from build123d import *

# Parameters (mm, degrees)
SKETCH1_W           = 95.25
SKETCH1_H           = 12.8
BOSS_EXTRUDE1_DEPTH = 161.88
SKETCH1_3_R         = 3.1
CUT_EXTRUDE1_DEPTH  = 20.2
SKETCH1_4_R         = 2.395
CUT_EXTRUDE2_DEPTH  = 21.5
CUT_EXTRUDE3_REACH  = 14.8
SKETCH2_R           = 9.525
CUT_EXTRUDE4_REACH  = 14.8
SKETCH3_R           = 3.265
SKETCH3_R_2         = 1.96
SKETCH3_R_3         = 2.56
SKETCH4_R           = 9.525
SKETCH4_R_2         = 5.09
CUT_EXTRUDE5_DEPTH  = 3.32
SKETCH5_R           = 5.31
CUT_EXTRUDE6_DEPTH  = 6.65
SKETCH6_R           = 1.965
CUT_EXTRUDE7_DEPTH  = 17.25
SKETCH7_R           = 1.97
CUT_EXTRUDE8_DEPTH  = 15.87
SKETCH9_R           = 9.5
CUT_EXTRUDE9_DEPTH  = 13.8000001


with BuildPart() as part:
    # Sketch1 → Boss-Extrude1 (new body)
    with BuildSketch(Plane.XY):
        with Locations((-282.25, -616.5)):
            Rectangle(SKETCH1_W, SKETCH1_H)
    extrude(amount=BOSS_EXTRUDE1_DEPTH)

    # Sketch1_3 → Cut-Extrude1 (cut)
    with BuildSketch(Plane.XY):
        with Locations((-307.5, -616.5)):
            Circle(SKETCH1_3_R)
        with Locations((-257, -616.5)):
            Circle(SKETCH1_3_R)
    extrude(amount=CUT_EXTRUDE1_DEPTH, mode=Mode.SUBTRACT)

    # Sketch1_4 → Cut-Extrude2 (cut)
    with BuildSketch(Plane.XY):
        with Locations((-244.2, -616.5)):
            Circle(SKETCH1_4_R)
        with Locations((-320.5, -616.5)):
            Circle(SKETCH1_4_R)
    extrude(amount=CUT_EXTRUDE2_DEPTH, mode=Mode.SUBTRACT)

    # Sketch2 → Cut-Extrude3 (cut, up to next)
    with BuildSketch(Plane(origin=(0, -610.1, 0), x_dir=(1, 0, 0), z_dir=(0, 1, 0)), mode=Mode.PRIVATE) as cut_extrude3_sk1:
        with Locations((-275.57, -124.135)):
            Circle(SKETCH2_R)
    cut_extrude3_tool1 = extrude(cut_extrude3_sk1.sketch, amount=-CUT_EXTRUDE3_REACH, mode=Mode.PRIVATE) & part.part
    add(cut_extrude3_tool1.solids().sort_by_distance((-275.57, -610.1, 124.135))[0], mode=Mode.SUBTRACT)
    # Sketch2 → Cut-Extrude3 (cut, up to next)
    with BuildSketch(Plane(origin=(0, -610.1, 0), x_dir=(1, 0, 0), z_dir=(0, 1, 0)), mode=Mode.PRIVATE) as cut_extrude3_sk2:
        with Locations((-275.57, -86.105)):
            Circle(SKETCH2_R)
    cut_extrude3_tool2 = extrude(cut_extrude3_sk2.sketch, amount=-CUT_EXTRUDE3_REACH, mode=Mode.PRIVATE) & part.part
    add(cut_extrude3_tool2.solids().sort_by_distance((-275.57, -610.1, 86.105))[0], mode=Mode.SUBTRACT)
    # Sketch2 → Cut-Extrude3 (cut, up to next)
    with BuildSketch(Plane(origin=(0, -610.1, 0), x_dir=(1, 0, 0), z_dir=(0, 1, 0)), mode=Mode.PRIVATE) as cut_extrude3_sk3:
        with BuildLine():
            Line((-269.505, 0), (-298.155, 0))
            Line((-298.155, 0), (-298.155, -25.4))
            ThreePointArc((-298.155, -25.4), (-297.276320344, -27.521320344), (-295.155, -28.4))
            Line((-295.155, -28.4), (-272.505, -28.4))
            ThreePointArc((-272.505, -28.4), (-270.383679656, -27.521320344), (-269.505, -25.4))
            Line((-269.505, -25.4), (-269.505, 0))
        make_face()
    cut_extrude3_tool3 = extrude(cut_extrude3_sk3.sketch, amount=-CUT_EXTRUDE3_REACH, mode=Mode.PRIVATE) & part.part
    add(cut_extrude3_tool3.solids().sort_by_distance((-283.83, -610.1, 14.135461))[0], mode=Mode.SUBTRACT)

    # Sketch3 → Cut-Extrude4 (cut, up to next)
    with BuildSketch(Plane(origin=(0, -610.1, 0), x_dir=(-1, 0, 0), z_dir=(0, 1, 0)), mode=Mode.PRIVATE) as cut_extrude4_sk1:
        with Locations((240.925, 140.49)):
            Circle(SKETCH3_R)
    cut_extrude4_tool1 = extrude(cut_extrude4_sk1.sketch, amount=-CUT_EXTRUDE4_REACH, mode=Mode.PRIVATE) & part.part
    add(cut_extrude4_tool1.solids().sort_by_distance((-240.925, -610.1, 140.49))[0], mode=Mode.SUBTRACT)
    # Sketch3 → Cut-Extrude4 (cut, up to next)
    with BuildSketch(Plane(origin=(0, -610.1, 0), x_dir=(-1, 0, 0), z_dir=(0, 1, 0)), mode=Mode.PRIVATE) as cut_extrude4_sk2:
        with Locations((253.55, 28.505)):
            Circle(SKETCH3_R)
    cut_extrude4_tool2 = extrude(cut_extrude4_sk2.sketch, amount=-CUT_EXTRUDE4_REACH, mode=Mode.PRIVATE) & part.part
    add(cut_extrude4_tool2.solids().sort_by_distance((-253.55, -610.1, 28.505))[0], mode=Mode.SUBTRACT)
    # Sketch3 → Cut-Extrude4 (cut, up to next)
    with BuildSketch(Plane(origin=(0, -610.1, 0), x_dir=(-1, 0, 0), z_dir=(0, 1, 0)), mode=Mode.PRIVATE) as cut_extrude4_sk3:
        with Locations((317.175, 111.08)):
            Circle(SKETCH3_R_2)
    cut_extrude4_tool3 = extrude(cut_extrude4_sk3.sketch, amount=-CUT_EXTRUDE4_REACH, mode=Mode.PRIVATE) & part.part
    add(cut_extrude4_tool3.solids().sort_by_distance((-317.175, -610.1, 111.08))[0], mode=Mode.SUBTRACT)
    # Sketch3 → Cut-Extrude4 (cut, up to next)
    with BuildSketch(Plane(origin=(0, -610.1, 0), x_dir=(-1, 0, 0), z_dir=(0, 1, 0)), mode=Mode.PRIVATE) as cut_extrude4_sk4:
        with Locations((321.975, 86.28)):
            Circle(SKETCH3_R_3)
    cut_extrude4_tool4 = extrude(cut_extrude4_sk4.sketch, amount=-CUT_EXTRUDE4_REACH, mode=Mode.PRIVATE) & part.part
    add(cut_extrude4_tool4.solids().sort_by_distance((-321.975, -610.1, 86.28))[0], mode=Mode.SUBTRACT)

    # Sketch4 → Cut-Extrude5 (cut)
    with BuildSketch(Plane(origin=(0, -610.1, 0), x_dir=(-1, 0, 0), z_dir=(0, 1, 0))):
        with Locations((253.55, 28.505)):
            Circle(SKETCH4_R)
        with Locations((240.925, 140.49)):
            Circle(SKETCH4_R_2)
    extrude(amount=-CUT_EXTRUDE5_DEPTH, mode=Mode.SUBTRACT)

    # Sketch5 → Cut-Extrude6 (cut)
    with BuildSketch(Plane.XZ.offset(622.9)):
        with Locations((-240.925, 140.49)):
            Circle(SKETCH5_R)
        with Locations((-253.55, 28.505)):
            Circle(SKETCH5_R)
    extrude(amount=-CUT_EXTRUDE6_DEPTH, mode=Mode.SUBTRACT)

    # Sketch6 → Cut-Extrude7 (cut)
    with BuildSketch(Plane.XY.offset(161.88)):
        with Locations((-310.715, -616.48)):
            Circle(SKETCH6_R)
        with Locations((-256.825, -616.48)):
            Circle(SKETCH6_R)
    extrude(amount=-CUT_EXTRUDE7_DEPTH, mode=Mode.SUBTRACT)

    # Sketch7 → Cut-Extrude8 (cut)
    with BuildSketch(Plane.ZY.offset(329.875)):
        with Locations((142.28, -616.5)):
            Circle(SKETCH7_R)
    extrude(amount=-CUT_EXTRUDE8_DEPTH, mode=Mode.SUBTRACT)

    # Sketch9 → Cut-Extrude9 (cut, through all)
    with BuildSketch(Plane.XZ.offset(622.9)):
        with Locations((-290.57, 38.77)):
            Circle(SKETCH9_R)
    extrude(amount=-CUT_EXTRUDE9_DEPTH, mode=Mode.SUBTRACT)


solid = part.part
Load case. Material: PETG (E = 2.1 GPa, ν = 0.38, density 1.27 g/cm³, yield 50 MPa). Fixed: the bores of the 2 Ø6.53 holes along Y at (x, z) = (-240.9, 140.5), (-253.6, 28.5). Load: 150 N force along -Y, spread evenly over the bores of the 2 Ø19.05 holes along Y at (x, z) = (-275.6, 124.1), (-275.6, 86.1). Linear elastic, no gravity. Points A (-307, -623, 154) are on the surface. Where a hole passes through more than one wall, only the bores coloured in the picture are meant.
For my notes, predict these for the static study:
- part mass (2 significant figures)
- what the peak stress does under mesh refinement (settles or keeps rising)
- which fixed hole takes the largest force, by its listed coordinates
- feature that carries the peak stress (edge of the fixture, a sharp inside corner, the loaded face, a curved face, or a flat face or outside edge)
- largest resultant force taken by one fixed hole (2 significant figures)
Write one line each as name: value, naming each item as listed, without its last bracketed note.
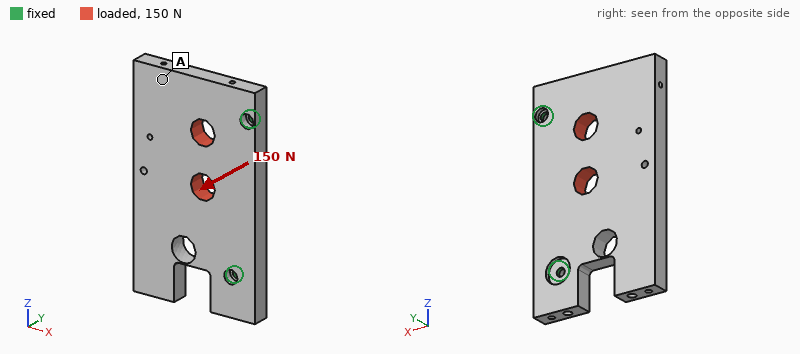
part mass: 220 g
what the peak stress does under mesh refinement: keeps rising
which fixed hole takes the largest force, by its listed coordinates: (-240.9, 140.5)
feature that carries the peak stress: edge of the fixture
largest resultant force taken by one fixed hole: 110 N
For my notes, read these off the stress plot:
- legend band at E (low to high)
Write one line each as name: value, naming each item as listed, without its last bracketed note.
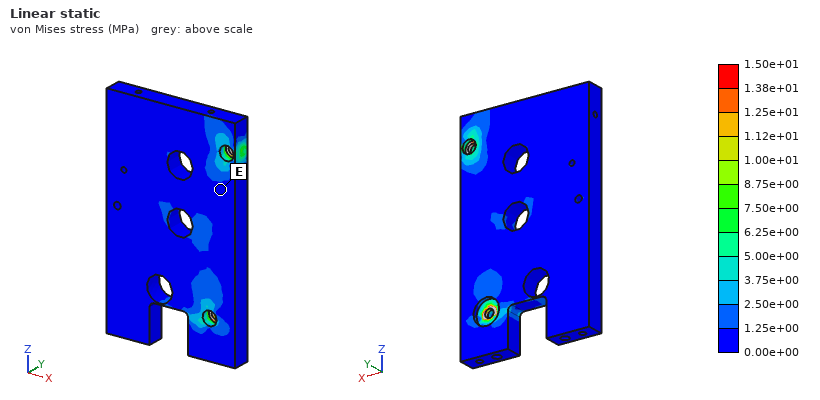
legend band at E: 0.00e+00 to 1.25e+00 MPa
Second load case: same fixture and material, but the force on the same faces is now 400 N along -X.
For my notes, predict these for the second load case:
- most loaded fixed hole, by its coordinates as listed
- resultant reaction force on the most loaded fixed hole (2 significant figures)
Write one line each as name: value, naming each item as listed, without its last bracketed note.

most loaded fixed hole, by its coordinates as listed: (-240.9, 140.5)
resultant reaction force on the most loaded fixed hole: 280 N
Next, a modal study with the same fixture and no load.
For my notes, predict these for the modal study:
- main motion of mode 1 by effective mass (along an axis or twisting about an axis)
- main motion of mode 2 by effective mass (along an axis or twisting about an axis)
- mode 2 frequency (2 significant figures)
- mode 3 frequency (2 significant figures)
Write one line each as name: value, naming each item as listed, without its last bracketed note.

main motion of mode 1 by effective mass: along Y
main motion of mode 2 by effective mass: twisting about X
mode 2 frequency: 360 Hz
mode 3 frequency: 670 Hz
